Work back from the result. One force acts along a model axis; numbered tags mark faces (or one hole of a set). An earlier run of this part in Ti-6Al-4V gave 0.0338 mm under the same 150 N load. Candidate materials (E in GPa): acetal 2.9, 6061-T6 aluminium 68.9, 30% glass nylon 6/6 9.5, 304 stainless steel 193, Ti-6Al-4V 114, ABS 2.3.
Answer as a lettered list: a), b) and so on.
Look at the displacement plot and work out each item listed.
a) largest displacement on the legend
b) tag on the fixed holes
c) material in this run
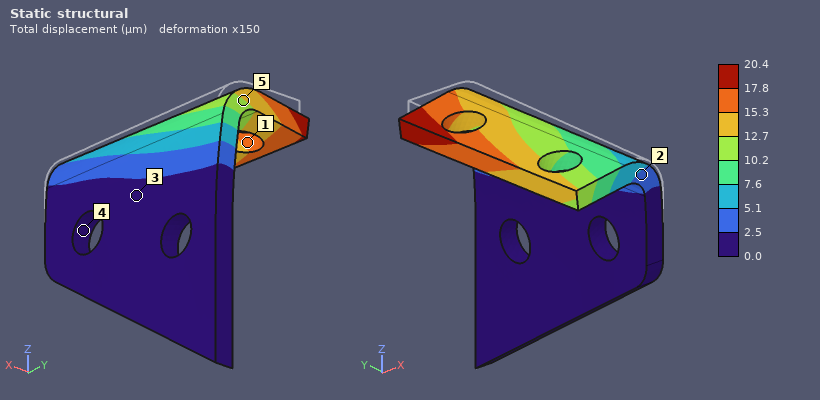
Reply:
a) 20.4 µm
b) 4
c) 304 stainless steel
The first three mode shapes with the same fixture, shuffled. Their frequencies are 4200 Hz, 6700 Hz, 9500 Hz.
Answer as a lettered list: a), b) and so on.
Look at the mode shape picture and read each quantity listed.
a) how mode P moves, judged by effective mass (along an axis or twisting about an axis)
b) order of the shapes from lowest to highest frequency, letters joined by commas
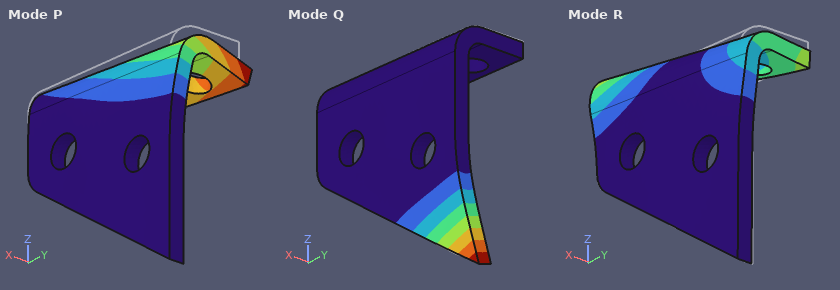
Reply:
a) along X
b) P, R, Q
